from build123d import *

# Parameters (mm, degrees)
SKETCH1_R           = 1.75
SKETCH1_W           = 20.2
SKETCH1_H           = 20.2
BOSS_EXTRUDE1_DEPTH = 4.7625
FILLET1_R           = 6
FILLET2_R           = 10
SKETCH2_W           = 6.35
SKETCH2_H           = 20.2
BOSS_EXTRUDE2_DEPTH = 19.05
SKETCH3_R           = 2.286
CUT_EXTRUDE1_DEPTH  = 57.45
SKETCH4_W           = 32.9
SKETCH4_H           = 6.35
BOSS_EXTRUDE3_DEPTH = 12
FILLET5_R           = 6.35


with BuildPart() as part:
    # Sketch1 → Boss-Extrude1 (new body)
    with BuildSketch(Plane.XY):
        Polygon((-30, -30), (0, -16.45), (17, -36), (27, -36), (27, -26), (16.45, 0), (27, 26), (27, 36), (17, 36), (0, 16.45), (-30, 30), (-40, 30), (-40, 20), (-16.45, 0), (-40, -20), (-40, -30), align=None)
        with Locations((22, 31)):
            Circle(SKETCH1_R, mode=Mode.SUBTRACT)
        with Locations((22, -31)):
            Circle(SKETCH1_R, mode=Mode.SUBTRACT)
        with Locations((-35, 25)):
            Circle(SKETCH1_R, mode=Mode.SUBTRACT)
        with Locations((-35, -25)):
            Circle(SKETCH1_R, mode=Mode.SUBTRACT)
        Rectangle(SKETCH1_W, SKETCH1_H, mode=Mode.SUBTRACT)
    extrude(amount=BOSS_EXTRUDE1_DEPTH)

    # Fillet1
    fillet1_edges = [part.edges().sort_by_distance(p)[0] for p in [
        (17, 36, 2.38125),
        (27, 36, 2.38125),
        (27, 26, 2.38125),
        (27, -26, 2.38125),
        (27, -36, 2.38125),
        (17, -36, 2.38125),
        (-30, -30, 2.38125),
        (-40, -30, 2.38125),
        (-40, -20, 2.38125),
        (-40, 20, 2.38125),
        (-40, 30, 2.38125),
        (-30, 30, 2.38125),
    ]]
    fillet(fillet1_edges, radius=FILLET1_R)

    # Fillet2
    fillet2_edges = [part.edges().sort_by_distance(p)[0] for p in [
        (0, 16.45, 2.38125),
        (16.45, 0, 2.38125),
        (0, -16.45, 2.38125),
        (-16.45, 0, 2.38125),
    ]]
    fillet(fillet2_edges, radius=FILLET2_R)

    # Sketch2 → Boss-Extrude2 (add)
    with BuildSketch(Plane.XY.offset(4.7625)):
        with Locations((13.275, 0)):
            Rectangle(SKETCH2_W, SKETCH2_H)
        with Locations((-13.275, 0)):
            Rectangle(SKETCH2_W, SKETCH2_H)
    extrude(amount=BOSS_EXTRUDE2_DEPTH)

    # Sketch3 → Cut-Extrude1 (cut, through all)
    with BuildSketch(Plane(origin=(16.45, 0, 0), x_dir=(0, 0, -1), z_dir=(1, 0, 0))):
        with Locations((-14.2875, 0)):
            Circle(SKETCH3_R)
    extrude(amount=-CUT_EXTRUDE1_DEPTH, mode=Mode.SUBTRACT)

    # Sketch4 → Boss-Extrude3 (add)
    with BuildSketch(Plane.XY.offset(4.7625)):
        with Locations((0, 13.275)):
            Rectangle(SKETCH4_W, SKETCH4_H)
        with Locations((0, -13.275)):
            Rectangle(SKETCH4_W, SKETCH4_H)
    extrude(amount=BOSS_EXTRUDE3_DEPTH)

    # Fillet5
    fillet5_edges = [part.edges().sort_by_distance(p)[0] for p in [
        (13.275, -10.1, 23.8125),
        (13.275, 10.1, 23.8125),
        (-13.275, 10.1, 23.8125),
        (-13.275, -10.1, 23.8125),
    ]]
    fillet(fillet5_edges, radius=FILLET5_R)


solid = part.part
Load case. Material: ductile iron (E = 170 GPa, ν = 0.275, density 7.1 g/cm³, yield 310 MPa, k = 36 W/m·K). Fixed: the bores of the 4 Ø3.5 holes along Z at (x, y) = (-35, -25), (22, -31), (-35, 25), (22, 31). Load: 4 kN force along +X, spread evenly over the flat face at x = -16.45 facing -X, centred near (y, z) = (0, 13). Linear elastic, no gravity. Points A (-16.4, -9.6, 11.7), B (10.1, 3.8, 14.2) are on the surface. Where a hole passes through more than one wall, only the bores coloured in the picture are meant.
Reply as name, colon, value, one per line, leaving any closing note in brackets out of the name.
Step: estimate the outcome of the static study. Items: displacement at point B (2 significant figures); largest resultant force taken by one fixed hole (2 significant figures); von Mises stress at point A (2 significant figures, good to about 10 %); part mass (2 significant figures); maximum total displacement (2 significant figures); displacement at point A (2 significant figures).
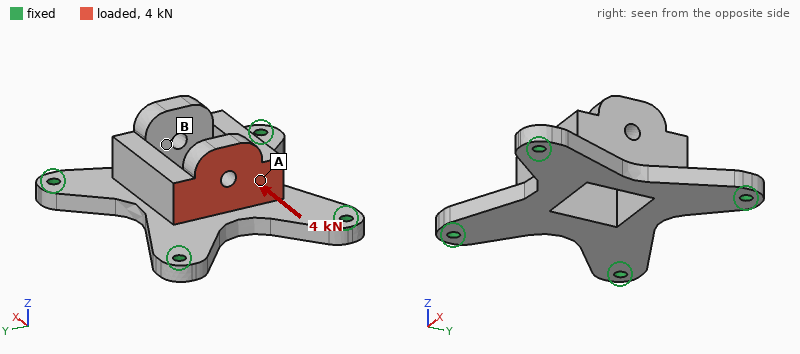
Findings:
displacement at point B: 15 µm
largest resultant force taken by one fixed hole: 1.5 kN
von Mises stress at point A: 49 MPa
part mass: 150 g
maximum total displacement: 42 µm
displacement at point A: 21 µm
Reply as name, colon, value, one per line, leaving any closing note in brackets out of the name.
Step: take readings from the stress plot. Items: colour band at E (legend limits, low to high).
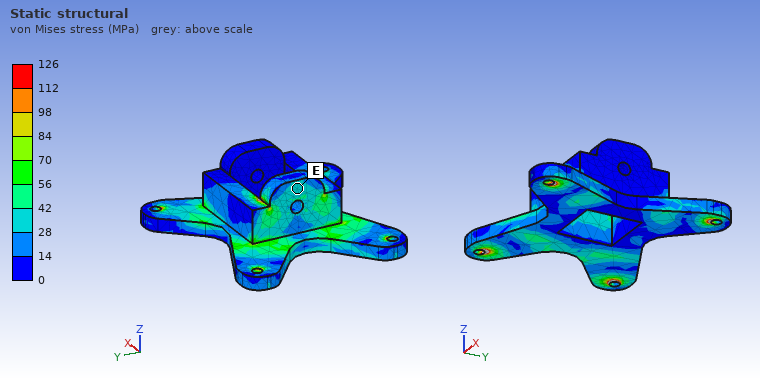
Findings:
colour band at E: 28 to 42 MPa
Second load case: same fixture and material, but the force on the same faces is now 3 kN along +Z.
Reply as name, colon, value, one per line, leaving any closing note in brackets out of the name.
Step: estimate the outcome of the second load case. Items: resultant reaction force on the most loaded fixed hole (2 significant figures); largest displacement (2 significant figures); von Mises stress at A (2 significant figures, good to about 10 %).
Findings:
resultant reaction force on the most loaded fixed hole: 1.2 kN
largest displacement: 64 µm
von Mises stress at A: 42 MPa
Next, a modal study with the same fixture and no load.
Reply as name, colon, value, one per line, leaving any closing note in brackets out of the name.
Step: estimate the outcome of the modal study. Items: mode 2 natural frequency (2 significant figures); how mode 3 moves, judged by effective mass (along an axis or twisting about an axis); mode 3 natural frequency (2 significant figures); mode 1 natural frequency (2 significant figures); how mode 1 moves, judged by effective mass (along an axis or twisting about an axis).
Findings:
mode 2 natural frequency: 6700 Hz
how mode 3 moves, judged by effective mass: along Y
mode 3 natural frequency: 7100 Hz
mode 1 natural frequency: 4500 Hz
how mode 1 moves, judged by effective mass: along Z
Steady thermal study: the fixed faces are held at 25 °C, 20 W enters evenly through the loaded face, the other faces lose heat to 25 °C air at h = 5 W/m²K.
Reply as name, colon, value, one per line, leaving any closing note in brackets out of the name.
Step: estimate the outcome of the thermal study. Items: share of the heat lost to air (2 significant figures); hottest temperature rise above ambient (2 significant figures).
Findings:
share of the heat lost to air: 7.1 %
hottest temperature rise above ambient: 74 K
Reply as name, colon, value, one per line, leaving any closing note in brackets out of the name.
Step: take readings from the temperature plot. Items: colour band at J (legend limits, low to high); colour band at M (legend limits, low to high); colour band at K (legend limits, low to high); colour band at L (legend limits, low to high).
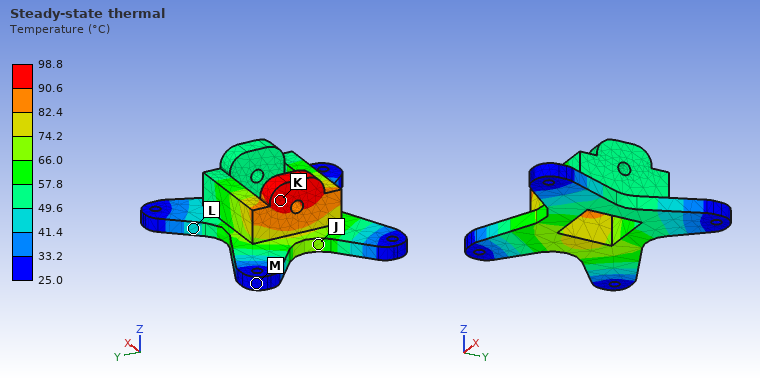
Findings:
colour band at J: 66.0 to 74.2 °C
colour band at M: 25.0 to 33.2 °C
colour band at K: 90.6 to 98.8 °C
colour band at L: 41.4 to 49.6 °C
